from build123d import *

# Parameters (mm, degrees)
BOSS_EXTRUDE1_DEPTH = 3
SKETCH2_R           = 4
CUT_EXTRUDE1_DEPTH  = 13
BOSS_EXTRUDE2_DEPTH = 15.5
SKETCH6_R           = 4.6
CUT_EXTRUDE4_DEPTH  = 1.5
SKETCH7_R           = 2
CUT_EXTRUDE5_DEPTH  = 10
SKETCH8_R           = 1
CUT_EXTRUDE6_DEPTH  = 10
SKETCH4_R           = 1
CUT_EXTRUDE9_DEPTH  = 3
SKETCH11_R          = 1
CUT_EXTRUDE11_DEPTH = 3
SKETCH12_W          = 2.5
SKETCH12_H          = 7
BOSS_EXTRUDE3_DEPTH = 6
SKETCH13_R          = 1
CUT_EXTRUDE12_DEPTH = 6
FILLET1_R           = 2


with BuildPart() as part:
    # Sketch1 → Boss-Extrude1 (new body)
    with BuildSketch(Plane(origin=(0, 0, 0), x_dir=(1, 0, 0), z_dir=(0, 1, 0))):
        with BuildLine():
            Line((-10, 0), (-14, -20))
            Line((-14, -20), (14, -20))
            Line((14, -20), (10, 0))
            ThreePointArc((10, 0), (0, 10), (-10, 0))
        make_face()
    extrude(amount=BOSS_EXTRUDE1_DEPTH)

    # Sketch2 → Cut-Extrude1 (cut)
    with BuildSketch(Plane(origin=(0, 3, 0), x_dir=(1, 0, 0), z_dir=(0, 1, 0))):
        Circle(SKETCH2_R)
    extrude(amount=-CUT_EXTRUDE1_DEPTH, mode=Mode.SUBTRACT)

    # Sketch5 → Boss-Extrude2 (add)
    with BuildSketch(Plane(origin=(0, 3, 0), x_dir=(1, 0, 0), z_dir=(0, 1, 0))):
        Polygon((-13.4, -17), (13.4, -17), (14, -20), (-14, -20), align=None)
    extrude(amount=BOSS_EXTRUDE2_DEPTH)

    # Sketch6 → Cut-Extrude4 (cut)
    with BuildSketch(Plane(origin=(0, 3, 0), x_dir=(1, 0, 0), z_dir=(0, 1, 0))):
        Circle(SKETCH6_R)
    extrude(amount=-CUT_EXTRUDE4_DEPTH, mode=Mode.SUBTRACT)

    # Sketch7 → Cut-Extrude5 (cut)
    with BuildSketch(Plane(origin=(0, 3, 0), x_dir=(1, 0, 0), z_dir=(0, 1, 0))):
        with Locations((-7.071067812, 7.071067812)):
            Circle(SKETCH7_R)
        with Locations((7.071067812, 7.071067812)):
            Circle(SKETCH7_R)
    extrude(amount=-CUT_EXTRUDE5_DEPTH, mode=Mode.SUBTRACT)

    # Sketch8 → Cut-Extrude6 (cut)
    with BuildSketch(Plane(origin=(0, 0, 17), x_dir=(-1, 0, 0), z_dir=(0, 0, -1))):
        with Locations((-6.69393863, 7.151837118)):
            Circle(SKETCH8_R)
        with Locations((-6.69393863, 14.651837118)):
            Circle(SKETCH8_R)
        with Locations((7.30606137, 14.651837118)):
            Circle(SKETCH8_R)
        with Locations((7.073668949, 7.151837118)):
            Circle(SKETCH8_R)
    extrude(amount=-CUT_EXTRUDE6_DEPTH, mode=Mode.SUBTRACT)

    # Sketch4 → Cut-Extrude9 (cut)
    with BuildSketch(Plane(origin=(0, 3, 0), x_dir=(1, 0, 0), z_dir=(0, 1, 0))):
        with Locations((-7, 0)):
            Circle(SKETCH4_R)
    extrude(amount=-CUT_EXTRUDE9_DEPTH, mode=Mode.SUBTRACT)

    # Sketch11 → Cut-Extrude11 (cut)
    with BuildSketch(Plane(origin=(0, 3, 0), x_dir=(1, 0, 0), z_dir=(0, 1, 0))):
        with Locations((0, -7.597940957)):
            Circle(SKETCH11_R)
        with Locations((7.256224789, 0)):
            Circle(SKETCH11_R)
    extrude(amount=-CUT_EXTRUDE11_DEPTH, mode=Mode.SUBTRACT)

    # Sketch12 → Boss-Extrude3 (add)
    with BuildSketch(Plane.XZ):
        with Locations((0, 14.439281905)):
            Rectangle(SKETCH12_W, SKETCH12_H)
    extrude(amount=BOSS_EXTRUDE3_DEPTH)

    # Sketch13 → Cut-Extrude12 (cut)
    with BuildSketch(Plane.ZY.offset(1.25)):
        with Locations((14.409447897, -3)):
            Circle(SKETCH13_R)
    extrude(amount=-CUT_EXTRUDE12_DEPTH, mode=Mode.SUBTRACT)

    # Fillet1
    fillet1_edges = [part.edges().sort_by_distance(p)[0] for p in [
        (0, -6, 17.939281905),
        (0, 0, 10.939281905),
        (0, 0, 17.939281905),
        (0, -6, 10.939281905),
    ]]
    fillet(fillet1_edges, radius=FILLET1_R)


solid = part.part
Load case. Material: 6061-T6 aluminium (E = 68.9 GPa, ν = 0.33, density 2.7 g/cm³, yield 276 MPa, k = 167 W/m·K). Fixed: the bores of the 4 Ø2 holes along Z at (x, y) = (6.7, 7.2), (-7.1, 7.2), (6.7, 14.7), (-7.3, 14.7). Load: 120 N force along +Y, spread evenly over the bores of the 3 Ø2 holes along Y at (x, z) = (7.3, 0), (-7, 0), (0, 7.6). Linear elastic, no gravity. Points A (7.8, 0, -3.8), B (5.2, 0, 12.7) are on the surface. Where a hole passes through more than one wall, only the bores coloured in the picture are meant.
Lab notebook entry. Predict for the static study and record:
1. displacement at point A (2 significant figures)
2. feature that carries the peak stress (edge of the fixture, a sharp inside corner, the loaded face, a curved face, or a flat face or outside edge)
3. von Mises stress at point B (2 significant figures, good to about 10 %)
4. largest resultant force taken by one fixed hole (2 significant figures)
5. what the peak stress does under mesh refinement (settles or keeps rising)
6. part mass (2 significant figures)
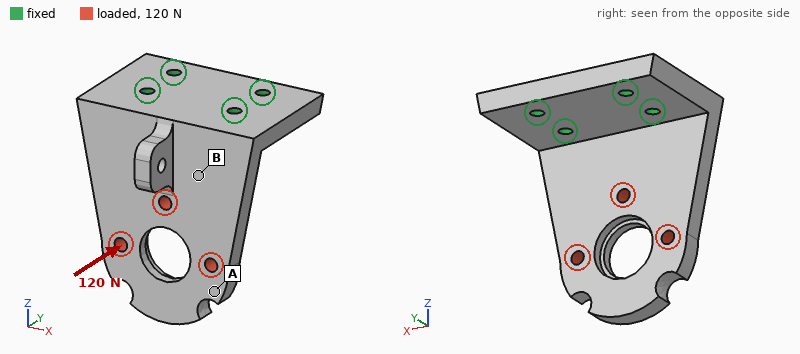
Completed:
0.11 mm
edge of the fixture
24 MPa
75 N
keeps rising
8.1 g
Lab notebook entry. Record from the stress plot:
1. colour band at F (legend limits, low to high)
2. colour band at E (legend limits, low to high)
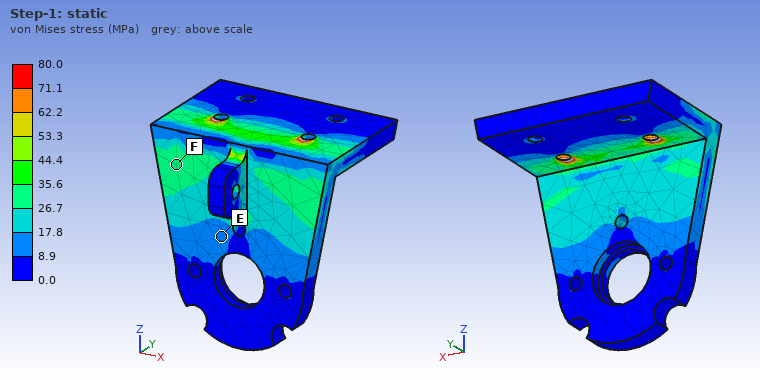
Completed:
26.7 to 35.6 MPa
8.9 to 17.8 MPa
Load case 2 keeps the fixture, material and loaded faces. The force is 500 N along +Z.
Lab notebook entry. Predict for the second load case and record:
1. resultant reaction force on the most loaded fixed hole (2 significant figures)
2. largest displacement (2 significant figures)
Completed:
320 N
65 µm
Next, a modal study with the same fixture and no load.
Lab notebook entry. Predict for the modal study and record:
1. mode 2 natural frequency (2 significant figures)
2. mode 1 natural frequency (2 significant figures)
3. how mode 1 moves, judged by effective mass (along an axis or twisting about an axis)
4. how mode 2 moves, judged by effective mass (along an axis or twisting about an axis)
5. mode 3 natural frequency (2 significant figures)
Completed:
8900 Hz
3400 Hz
along Y
along X
12 kHz
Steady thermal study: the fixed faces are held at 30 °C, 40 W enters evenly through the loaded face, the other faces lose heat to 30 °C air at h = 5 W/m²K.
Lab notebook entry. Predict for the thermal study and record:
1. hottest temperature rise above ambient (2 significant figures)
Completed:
82 K
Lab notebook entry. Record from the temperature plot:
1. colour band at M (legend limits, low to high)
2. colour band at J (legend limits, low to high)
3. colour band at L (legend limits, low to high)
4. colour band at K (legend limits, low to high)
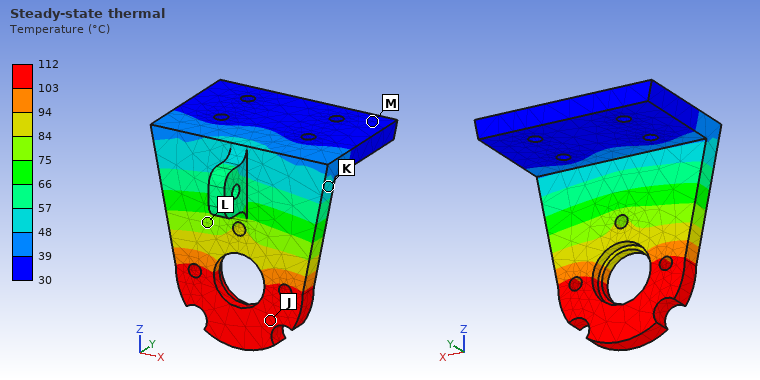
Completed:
30 to 39 °C
103 to 112 °C
75 to 84 °C
48 to 57 °C
